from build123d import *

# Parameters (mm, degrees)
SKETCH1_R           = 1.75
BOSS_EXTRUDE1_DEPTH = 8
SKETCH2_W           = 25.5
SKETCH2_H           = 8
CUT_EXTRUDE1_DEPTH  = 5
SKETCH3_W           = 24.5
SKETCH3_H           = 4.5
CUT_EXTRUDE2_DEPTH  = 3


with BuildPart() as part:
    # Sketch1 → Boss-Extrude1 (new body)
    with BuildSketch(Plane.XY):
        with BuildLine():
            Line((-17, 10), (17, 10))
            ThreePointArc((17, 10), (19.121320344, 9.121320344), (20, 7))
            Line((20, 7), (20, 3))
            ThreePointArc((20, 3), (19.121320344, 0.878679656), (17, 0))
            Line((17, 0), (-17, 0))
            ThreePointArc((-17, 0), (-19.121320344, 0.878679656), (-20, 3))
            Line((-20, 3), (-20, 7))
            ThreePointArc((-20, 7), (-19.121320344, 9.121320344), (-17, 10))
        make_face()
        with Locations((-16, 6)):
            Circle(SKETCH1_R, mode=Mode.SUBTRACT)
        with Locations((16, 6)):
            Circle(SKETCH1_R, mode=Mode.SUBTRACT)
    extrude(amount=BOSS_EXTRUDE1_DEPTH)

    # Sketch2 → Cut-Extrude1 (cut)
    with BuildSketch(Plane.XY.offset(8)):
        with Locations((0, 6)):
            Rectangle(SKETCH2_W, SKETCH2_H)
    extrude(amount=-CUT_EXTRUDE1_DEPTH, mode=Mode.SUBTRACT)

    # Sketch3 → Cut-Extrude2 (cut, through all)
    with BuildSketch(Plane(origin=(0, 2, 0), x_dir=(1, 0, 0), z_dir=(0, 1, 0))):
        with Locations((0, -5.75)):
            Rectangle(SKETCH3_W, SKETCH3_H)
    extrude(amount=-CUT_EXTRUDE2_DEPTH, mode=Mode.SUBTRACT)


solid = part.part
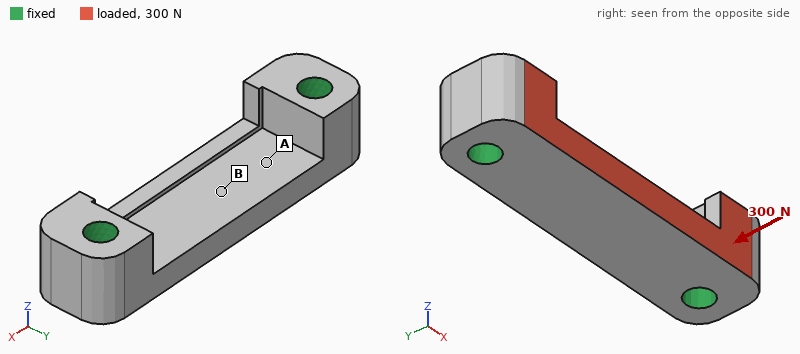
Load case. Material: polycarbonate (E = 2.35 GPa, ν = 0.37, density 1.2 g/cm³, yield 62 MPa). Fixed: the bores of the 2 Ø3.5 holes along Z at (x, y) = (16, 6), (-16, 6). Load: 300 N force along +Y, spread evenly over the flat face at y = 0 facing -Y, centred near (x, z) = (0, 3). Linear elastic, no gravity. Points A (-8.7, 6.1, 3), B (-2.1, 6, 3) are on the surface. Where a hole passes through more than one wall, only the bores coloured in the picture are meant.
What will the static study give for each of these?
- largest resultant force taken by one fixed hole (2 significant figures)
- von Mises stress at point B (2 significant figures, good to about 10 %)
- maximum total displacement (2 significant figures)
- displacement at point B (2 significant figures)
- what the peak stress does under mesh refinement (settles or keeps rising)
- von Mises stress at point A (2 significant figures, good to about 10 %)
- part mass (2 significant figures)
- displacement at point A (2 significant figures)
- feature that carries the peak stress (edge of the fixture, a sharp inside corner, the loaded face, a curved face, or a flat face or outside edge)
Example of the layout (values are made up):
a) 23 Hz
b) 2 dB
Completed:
a) 150 N
b) 1.8 MPa
c) 77 µm
d) 69 µm
e) keeps rising
f) 5.7 MPa
g) 2.1 g
h) 40 µm
i) edge of the fixture
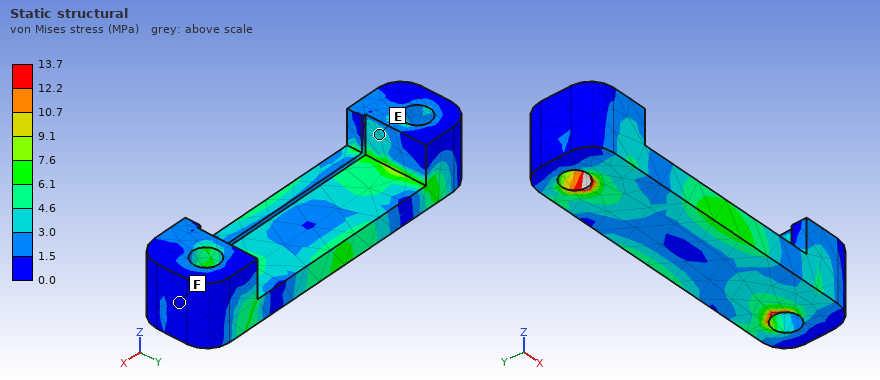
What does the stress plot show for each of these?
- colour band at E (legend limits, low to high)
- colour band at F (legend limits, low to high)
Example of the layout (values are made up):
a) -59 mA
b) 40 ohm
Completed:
a) 3.0 to 4.6 MPa
b) 0.0 to 1.5 MPa
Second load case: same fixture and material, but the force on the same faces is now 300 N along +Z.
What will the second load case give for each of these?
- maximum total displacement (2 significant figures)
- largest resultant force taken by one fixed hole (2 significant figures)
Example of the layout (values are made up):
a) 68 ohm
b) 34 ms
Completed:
a) 0.40 mm
b) 150 N
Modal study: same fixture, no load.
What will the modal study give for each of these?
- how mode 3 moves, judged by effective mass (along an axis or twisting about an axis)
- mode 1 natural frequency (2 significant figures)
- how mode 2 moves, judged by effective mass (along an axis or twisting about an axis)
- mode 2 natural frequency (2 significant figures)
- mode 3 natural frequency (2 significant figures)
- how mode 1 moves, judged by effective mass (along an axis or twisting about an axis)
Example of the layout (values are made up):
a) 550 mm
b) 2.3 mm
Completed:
a) along Y
b) 5400 Hz
c) along Y
d) 8800 Hz
e) 9300 Hz
f) along Z
